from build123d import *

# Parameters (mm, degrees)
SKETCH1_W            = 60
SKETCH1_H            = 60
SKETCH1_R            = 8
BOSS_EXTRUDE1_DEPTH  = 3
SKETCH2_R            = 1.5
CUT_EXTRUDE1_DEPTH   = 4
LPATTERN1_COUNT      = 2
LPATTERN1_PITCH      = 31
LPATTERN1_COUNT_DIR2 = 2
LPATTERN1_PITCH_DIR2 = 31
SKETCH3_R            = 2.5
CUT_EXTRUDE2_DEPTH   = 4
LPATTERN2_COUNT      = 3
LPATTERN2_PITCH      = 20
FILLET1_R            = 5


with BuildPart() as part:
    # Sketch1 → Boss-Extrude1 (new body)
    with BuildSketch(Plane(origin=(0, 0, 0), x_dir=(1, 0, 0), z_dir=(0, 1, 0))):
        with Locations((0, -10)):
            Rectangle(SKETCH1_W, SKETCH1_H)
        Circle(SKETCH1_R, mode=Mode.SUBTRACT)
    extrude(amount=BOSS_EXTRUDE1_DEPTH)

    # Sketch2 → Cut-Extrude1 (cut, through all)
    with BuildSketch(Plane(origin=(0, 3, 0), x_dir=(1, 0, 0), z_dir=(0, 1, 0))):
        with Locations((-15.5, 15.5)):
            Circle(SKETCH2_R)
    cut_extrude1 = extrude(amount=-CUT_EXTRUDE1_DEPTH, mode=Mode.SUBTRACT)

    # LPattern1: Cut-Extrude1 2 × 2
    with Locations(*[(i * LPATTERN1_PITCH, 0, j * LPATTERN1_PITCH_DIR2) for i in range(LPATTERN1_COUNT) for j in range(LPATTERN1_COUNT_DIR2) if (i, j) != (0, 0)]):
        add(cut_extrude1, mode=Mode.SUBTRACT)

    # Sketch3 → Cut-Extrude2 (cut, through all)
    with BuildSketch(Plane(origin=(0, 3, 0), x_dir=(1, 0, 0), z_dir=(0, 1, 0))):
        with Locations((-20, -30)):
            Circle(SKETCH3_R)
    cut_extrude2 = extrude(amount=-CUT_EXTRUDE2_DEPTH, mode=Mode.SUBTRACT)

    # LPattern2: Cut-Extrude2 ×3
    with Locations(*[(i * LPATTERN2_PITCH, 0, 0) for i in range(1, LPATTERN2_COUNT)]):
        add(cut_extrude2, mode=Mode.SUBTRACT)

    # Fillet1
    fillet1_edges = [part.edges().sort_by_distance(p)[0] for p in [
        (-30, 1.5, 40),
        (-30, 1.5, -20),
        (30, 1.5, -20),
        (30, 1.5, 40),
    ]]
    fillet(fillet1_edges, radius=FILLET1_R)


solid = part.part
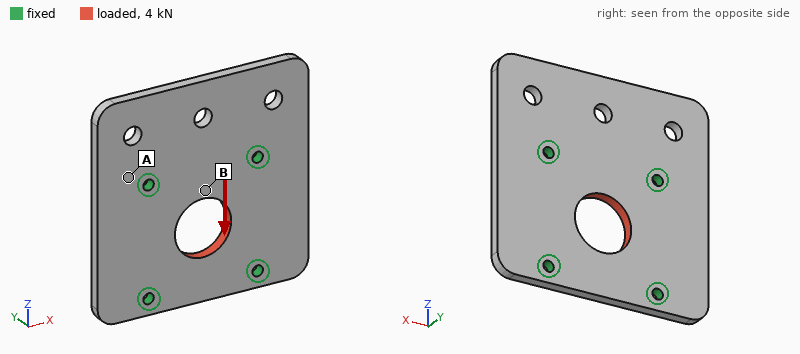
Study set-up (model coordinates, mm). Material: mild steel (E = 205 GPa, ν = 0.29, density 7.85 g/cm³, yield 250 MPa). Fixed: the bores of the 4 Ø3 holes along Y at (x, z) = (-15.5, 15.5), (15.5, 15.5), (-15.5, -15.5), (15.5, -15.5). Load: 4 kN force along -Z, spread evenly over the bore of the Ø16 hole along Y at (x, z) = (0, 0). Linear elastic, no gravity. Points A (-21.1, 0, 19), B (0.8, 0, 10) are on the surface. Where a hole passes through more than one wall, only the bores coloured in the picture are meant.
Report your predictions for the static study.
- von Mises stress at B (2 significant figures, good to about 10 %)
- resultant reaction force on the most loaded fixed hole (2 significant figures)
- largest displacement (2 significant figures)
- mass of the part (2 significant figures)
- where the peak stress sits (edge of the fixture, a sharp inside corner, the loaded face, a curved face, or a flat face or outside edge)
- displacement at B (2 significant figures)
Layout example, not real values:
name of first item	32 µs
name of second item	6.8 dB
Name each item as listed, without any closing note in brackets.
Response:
von Mises stress at B	24 MPa
resultant reaction force on the most loaded fixed hole	1.1 kN
largest displacement	4.0 µm
mass of the part	77 g
where the peak stress sits	edge of the fixture
displacement at B	2.4 µm
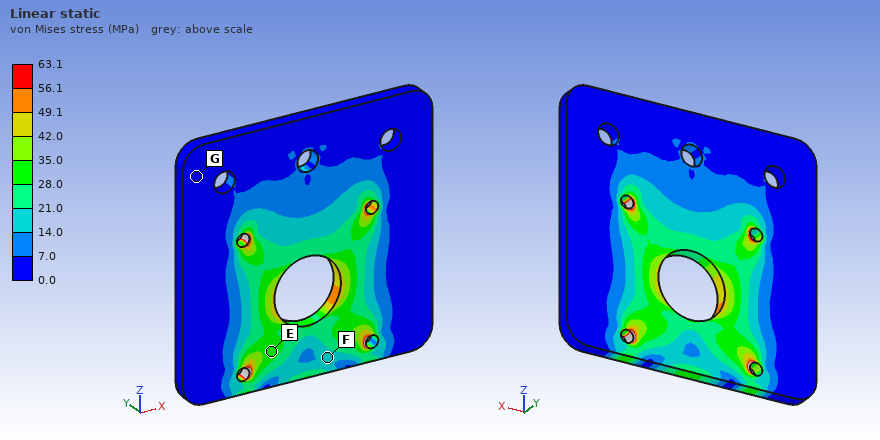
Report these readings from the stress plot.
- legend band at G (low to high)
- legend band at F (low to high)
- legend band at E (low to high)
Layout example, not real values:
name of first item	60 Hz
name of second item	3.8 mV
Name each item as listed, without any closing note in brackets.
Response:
legend band at G	0.0 to 7.0 MPa
legend band at F	14.0 to 21.0 MPa
legend band at E	28.0 to 35.0 MPa
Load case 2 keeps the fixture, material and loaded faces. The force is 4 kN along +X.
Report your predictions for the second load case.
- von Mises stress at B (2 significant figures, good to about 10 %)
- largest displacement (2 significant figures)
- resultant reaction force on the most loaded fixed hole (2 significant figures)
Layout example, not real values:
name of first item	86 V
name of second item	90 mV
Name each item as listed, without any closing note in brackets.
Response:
von Mises stress at B	33 MPa
largest displacement	2.9 µm
resultant reaction force on the most loaded fixed hole	1.0 kN
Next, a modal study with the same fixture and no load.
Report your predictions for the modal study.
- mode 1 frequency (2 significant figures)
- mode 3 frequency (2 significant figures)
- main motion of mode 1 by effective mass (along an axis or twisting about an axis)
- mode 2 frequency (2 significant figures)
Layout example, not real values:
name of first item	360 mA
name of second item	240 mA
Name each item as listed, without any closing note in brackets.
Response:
mode 1 frequency	3700 Hz
mode 3 frequency	7300 Hz
main motion of mode 1 by effective mass	along Y
mode 2 frequency	5000 Hz
